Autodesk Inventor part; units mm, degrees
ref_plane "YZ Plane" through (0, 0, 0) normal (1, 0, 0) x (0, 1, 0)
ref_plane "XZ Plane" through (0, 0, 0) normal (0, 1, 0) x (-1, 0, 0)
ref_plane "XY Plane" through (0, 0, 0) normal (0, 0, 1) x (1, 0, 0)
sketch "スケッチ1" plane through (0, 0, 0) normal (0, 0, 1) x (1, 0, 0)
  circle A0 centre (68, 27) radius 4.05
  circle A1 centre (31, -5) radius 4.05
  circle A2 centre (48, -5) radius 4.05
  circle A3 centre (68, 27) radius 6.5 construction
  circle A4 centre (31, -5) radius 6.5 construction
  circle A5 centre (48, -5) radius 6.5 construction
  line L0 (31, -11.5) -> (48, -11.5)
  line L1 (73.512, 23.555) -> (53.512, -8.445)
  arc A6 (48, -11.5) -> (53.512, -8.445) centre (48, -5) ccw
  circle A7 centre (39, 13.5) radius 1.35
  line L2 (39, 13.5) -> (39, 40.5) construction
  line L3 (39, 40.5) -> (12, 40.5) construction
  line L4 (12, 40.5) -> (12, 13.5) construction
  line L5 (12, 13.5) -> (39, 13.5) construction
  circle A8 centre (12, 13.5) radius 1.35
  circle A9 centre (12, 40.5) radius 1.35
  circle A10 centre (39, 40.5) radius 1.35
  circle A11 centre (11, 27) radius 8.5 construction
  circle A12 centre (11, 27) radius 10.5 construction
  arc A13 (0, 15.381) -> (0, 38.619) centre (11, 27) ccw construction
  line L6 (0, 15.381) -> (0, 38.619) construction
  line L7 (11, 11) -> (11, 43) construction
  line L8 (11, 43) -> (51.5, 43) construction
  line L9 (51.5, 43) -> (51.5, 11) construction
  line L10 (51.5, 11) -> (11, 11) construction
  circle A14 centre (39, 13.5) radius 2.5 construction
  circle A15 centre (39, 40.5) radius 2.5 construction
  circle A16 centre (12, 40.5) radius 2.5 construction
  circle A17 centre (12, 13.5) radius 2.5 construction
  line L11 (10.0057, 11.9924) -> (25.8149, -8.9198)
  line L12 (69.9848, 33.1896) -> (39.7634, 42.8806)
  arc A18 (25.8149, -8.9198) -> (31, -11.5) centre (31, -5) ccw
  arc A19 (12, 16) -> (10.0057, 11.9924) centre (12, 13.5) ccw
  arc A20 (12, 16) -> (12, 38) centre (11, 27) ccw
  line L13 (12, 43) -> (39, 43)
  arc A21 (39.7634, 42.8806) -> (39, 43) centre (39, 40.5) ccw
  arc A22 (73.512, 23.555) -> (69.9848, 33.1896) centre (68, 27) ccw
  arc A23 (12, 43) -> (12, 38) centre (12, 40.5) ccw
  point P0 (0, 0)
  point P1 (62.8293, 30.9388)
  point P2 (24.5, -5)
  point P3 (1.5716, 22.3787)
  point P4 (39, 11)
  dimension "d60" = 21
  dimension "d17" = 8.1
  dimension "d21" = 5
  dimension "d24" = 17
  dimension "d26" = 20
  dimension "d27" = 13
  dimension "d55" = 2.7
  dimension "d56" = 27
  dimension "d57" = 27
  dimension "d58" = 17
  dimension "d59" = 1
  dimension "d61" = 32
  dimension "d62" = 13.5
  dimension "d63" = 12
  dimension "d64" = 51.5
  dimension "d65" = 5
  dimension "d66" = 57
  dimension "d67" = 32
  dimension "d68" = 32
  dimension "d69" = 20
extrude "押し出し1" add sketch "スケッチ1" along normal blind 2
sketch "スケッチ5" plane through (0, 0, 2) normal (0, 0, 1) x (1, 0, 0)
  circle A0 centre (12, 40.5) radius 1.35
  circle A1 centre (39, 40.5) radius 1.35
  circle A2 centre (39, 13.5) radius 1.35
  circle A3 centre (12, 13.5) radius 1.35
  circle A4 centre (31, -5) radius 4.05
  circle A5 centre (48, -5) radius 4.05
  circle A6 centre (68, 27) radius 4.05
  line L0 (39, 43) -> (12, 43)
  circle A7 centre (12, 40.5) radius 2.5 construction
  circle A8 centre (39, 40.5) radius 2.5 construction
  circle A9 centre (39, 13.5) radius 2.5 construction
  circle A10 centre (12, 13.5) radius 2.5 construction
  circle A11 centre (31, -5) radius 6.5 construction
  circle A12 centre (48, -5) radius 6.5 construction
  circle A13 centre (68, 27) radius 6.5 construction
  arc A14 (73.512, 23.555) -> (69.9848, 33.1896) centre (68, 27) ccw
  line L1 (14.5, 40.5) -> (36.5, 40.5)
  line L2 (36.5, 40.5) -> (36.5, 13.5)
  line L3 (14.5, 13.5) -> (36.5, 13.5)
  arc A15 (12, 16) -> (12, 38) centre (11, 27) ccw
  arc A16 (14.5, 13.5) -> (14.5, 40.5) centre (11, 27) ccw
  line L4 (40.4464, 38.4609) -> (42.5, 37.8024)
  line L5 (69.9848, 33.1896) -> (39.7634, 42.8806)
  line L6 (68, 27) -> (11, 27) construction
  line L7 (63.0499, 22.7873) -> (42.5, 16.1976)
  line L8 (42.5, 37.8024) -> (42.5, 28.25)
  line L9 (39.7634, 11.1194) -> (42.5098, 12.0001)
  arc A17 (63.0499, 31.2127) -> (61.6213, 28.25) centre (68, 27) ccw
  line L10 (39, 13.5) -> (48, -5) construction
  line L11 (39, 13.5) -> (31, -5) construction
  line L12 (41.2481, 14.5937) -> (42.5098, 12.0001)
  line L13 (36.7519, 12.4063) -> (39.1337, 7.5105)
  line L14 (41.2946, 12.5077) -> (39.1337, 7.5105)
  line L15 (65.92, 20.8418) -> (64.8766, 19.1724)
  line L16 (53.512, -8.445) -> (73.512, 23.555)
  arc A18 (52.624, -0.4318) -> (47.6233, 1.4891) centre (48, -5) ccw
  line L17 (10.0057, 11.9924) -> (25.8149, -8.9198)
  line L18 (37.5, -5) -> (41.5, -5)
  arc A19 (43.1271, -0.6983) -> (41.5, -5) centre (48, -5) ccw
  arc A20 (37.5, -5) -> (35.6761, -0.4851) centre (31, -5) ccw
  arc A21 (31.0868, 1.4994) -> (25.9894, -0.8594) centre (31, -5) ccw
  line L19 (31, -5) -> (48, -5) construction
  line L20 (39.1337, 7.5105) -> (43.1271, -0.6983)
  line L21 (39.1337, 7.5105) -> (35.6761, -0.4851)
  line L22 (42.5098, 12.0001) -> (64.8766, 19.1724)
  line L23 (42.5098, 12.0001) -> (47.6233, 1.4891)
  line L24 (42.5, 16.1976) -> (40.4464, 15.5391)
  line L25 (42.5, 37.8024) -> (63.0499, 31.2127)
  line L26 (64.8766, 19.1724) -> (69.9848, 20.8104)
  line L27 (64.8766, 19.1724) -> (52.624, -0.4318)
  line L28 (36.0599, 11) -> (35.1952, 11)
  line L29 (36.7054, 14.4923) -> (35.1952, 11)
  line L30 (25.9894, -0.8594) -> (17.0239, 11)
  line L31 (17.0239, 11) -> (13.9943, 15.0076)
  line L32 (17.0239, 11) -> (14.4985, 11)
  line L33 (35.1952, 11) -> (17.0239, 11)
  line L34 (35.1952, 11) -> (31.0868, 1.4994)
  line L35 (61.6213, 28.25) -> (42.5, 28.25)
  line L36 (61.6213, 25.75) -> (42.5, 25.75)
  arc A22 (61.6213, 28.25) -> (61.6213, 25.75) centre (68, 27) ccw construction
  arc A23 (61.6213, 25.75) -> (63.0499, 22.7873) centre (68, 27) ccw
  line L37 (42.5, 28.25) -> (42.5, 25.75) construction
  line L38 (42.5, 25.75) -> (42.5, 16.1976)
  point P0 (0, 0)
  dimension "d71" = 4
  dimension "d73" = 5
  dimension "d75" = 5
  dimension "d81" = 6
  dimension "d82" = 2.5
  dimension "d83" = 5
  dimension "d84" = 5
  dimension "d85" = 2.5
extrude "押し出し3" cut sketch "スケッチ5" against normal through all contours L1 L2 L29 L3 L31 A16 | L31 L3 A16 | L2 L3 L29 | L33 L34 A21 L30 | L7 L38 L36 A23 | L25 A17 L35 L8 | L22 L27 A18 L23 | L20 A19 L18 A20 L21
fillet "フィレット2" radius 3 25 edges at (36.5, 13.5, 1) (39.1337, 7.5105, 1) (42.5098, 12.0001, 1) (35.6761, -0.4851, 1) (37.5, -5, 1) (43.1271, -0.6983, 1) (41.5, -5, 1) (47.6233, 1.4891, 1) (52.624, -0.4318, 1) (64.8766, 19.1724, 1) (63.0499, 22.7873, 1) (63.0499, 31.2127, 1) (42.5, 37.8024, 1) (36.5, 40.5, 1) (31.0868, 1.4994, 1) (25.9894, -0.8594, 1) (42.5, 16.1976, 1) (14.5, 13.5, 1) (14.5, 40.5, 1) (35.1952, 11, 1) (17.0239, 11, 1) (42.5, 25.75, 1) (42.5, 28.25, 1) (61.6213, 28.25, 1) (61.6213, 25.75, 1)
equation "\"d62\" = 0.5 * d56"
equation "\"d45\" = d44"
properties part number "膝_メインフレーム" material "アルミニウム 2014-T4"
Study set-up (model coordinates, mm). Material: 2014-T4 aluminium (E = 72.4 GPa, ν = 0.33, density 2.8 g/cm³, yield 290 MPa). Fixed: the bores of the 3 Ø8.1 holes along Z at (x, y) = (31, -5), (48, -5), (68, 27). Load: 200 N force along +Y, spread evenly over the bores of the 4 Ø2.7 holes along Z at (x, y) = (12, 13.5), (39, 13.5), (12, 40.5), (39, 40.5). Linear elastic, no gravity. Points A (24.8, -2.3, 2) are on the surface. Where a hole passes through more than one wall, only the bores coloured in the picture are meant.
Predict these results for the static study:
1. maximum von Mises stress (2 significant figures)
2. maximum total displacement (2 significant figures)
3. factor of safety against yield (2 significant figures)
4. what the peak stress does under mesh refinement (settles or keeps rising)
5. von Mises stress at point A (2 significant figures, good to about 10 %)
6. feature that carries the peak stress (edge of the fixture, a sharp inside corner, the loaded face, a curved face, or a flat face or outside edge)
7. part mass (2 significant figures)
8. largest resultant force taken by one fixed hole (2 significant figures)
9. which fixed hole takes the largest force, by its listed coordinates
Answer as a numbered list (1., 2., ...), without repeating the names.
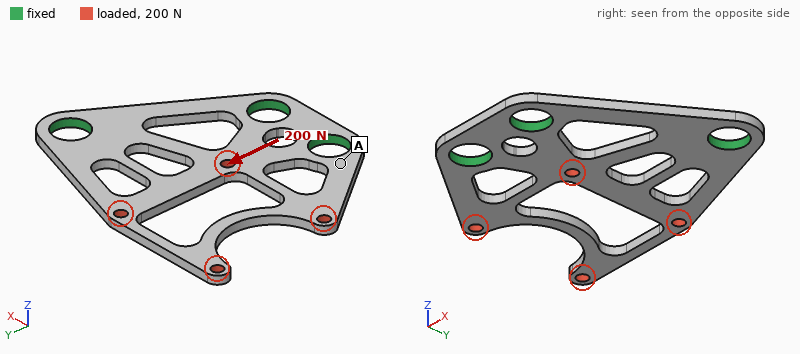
1. 90 MPa
2. 80 µm
3. 3.2
4. settles
5. 12 MPa
6. a curved face
7. 8.0 g
8. 150 N
9. (31, -5)
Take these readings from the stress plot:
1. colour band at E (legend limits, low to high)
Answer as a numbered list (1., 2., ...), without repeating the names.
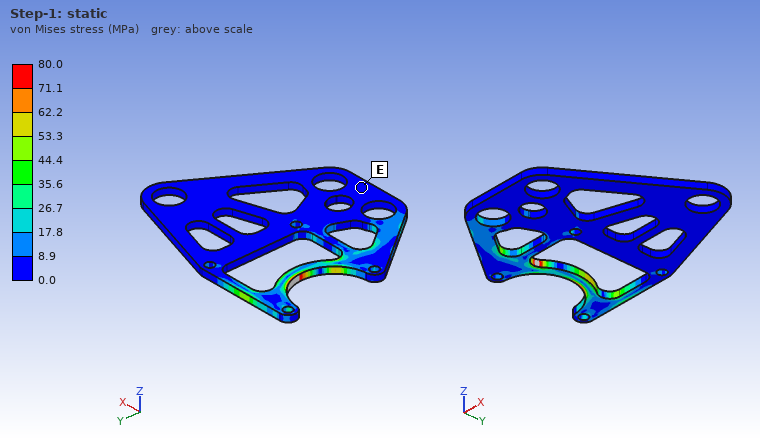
1. 0.0 to 8.9 MPa
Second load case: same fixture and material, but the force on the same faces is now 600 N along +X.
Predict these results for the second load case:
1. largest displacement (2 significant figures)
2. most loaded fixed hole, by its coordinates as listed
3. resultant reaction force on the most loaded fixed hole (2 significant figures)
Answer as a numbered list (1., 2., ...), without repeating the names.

1. 36 µm
2. (68, 27)
3. 440 N
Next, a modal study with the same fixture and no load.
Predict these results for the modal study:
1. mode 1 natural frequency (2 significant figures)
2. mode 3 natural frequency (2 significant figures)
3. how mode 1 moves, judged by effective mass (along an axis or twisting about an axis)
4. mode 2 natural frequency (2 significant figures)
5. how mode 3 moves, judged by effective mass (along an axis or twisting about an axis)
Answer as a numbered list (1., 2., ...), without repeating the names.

1. 1100 Hz
2. 3400 Hz
3. along Z
4. 3100 Hz
5. along Z
